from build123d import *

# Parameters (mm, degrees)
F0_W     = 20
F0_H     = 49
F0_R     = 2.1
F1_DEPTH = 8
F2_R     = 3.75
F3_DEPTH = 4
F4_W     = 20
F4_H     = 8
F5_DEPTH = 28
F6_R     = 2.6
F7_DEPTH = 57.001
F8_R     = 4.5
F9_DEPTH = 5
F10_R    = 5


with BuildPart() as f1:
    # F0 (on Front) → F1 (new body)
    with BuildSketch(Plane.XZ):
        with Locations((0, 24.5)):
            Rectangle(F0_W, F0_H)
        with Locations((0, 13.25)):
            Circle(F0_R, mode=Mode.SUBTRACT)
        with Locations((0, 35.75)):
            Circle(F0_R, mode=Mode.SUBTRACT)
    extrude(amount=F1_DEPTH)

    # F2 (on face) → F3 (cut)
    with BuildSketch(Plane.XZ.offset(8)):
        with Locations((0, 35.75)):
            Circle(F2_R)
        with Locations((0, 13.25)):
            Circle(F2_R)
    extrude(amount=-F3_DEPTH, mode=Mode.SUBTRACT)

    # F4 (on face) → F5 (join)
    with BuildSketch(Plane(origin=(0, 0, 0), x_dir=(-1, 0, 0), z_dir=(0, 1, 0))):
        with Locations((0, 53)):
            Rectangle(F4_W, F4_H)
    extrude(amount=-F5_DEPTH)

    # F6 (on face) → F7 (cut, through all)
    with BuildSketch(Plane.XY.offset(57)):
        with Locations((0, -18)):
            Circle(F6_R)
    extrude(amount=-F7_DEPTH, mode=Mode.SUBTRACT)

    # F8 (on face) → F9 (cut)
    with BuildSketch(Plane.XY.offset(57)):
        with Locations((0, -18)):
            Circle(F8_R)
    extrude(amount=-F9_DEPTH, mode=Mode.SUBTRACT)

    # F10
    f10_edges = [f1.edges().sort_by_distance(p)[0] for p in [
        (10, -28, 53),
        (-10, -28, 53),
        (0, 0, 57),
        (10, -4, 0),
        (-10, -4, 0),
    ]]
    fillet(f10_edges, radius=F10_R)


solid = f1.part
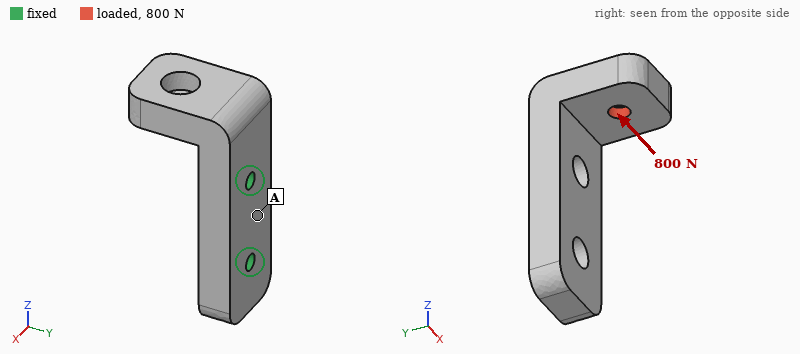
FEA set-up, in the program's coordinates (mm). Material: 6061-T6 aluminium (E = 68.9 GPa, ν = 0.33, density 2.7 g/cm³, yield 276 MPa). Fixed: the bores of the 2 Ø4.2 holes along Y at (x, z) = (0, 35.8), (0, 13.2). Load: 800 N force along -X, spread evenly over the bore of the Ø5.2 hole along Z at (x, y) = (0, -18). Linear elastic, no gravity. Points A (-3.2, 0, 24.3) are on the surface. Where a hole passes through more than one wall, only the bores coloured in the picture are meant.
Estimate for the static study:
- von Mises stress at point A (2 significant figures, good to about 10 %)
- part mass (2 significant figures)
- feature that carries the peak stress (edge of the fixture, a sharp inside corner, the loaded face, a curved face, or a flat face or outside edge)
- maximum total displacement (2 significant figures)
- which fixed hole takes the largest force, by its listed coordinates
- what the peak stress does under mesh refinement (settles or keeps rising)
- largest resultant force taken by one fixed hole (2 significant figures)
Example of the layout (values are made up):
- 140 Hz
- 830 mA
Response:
- 25 MPa
- 30 g
- edge of the fixture
- 0.14 mm
- (0, 35.8)
- keeps rising
- 1.1 kN
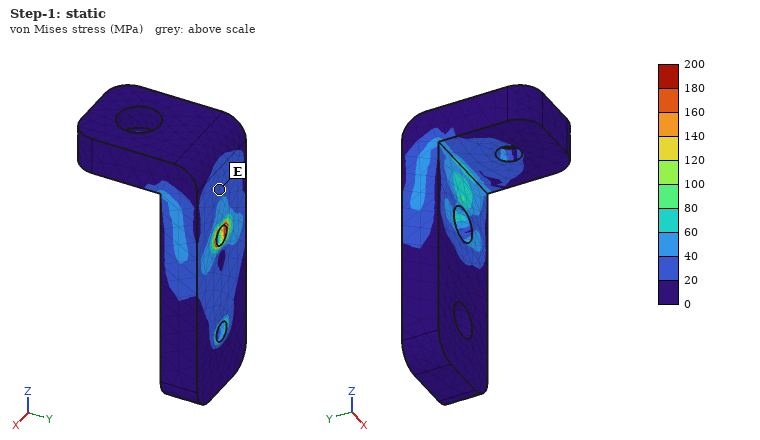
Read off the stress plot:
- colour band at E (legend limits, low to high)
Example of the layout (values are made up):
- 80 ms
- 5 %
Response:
- 20 to 40 MPa
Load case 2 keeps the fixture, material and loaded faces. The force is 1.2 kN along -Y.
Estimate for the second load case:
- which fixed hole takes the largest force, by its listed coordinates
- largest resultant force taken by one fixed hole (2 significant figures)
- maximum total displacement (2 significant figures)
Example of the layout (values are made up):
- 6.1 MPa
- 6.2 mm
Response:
- (0, 35.8)
- 1.9 kN
- 0.11 mm
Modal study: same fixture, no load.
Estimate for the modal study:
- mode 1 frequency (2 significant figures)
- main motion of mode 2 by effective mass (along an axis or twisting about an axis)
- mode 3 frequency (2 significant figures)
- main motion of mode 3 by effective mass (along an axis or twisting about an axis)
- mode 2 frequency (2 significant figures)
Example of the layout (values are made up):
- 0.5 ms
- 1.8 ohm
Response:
- 4300 Hz
- along X
- 12 kHz
- along Y
- 4900 Hz
